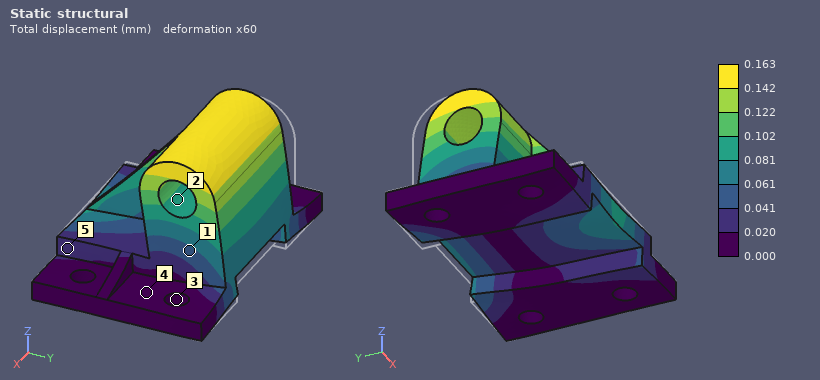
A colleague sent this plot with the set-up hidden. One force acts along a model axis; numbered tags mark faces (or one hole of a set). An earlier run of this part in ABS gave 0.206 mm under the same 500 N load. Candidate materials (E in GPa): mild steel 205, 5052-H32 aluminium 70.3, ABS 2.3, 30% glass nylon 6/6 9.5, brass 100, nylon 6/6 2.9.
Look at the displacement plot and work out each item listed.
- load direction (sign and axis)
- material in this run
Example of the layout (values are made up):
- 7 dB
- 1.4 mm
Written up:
- -Y
- nylon 6/6
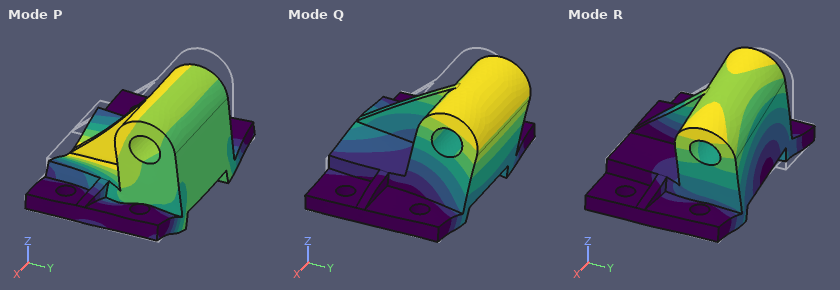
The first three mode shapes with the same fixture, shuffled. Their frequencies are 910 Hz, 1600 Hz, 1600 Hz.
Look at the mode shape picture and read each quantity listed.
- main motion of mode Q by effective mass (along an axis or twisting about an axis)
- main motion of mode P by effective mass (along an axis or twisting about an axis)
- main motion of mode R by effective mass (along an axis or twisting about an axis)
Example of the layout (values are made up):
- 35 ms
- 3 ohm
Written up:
- along Y
- along Z
- along X
